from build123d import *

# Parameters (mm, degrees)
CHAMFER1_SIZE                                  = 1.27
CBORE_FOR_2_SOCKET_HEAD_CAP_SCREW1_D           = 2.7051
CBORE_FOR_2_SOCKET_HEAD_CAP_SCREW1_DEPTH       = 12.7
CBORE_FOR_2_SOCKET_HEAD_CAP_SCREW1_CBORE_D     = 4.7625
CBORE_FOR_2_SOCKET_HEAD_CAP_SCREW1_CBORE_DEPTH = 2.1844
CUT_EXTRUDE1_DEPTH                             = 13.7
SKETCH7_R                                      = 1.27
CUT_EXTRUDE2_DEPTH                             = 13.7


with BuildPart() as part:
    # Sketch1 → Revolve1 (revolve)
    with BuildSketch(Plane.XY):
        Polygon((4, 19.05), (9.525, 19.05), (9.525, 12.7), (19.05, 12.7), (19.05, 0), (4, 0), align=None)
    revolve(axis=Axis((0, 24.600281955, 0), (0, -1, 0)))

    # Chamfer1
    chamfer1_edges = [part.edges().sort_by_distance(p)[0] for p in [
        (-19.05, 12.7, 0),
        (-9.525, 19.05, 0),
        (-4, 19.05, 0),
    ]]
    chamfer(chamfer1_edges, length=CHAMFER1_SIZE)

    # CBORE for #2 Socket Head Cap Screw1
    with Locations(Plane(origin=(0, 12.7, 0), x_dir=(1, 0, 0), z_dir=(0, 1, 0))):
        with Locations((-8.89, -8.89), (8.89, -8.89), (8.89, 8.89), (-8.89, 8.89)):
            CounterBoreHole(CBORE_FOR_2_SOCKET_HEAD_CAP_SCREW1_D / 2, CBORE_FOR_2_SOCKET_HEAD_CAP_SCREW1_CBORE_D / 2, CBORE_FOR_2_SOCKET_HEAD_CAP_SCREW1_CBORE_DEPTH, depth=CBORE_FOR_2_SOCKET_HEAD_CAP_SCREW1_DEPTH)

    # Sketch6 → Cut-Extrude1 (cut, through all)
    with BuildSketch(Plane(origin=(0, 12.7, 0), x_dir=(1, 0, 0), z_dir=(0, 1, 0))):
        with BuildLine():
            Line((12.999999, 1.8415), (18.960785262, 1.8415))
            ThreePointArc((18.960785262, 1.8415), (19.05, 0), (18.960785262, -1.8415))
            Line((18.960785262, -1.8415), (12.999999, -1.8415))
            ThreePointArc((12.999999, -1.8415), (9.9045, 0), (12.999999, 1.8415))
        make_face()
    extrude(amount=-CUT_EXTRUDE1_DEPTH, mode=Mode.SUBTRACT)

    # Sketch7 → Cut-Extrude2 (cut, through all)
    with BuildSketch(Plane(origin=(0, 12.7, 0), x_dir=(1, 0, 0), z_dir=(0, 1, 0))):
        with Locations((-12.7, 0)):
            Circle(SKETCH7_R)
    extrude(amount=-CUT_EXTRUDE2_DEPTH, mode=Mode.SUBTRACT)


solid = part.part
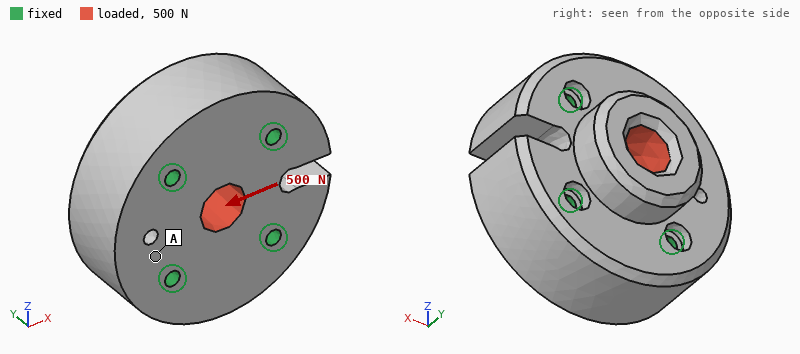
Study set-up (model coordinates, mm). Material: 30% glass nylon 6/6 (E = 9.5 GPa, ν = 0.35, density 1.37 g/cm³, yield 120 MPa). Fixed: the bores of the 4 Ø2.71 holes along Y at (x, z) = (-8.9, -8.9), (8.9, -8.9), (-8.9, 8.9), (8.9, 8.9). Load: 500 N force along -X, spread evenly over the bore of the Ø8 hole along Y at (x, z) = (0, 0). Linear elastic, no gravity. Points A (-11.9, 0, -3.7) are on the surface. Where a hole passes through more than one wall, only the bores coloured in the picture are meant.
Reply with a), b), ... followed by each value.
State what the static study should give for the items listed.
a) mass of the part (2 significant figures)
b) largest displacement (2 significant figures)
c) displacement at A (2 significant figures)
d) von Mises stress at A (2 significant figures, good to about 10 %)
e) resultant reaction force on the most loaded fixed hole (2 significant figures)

a) 20 g
b) 3.3 µm
c) 0.69 µm
d) 0.53 MPa
e) 140 N
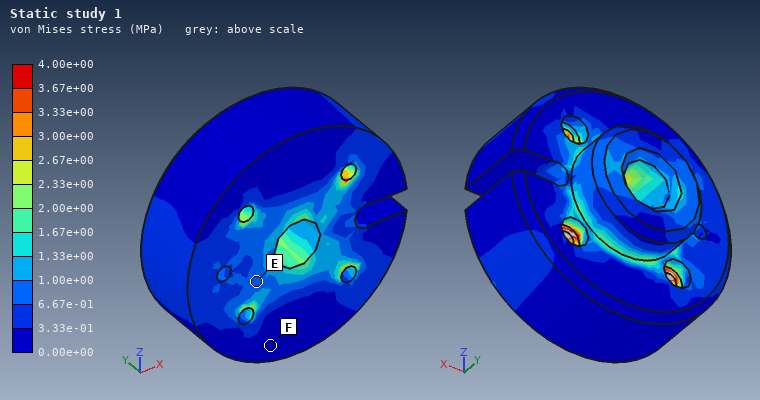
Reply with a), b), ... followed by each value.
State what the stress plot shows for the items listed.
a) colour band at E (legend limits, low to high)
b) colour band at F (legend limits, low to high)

a) 6.67e-01 to 1.00e+00 MPa
b) 0.00e+00 to 3.33e-01 MPa
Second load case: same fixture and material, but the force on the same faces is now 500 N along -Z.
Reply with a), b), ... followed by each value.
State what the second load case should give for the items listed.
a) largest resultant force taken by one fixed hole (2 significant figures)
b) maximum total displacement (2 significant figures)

a) 130 N
b) 3.0 µm
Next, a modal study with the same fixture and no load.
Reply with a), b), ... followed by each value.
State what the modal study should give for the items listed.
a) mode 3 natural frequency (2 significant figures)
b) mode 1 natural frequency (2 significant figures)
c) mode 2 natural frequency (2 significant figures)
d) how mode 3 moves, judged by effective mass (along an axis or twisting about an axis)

a) 25 kHz
b) 23 kHz
c) 23 kHz
d) along Y
